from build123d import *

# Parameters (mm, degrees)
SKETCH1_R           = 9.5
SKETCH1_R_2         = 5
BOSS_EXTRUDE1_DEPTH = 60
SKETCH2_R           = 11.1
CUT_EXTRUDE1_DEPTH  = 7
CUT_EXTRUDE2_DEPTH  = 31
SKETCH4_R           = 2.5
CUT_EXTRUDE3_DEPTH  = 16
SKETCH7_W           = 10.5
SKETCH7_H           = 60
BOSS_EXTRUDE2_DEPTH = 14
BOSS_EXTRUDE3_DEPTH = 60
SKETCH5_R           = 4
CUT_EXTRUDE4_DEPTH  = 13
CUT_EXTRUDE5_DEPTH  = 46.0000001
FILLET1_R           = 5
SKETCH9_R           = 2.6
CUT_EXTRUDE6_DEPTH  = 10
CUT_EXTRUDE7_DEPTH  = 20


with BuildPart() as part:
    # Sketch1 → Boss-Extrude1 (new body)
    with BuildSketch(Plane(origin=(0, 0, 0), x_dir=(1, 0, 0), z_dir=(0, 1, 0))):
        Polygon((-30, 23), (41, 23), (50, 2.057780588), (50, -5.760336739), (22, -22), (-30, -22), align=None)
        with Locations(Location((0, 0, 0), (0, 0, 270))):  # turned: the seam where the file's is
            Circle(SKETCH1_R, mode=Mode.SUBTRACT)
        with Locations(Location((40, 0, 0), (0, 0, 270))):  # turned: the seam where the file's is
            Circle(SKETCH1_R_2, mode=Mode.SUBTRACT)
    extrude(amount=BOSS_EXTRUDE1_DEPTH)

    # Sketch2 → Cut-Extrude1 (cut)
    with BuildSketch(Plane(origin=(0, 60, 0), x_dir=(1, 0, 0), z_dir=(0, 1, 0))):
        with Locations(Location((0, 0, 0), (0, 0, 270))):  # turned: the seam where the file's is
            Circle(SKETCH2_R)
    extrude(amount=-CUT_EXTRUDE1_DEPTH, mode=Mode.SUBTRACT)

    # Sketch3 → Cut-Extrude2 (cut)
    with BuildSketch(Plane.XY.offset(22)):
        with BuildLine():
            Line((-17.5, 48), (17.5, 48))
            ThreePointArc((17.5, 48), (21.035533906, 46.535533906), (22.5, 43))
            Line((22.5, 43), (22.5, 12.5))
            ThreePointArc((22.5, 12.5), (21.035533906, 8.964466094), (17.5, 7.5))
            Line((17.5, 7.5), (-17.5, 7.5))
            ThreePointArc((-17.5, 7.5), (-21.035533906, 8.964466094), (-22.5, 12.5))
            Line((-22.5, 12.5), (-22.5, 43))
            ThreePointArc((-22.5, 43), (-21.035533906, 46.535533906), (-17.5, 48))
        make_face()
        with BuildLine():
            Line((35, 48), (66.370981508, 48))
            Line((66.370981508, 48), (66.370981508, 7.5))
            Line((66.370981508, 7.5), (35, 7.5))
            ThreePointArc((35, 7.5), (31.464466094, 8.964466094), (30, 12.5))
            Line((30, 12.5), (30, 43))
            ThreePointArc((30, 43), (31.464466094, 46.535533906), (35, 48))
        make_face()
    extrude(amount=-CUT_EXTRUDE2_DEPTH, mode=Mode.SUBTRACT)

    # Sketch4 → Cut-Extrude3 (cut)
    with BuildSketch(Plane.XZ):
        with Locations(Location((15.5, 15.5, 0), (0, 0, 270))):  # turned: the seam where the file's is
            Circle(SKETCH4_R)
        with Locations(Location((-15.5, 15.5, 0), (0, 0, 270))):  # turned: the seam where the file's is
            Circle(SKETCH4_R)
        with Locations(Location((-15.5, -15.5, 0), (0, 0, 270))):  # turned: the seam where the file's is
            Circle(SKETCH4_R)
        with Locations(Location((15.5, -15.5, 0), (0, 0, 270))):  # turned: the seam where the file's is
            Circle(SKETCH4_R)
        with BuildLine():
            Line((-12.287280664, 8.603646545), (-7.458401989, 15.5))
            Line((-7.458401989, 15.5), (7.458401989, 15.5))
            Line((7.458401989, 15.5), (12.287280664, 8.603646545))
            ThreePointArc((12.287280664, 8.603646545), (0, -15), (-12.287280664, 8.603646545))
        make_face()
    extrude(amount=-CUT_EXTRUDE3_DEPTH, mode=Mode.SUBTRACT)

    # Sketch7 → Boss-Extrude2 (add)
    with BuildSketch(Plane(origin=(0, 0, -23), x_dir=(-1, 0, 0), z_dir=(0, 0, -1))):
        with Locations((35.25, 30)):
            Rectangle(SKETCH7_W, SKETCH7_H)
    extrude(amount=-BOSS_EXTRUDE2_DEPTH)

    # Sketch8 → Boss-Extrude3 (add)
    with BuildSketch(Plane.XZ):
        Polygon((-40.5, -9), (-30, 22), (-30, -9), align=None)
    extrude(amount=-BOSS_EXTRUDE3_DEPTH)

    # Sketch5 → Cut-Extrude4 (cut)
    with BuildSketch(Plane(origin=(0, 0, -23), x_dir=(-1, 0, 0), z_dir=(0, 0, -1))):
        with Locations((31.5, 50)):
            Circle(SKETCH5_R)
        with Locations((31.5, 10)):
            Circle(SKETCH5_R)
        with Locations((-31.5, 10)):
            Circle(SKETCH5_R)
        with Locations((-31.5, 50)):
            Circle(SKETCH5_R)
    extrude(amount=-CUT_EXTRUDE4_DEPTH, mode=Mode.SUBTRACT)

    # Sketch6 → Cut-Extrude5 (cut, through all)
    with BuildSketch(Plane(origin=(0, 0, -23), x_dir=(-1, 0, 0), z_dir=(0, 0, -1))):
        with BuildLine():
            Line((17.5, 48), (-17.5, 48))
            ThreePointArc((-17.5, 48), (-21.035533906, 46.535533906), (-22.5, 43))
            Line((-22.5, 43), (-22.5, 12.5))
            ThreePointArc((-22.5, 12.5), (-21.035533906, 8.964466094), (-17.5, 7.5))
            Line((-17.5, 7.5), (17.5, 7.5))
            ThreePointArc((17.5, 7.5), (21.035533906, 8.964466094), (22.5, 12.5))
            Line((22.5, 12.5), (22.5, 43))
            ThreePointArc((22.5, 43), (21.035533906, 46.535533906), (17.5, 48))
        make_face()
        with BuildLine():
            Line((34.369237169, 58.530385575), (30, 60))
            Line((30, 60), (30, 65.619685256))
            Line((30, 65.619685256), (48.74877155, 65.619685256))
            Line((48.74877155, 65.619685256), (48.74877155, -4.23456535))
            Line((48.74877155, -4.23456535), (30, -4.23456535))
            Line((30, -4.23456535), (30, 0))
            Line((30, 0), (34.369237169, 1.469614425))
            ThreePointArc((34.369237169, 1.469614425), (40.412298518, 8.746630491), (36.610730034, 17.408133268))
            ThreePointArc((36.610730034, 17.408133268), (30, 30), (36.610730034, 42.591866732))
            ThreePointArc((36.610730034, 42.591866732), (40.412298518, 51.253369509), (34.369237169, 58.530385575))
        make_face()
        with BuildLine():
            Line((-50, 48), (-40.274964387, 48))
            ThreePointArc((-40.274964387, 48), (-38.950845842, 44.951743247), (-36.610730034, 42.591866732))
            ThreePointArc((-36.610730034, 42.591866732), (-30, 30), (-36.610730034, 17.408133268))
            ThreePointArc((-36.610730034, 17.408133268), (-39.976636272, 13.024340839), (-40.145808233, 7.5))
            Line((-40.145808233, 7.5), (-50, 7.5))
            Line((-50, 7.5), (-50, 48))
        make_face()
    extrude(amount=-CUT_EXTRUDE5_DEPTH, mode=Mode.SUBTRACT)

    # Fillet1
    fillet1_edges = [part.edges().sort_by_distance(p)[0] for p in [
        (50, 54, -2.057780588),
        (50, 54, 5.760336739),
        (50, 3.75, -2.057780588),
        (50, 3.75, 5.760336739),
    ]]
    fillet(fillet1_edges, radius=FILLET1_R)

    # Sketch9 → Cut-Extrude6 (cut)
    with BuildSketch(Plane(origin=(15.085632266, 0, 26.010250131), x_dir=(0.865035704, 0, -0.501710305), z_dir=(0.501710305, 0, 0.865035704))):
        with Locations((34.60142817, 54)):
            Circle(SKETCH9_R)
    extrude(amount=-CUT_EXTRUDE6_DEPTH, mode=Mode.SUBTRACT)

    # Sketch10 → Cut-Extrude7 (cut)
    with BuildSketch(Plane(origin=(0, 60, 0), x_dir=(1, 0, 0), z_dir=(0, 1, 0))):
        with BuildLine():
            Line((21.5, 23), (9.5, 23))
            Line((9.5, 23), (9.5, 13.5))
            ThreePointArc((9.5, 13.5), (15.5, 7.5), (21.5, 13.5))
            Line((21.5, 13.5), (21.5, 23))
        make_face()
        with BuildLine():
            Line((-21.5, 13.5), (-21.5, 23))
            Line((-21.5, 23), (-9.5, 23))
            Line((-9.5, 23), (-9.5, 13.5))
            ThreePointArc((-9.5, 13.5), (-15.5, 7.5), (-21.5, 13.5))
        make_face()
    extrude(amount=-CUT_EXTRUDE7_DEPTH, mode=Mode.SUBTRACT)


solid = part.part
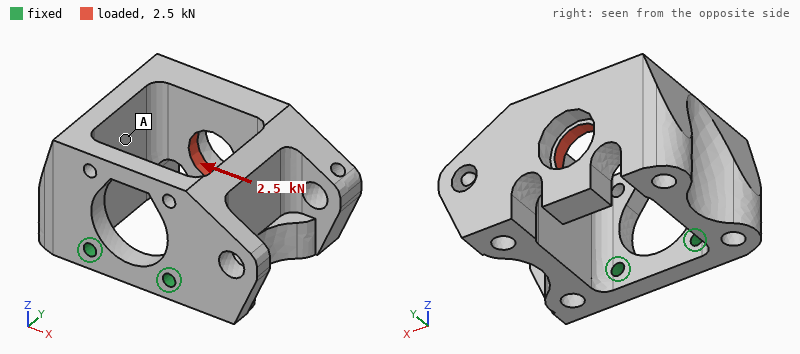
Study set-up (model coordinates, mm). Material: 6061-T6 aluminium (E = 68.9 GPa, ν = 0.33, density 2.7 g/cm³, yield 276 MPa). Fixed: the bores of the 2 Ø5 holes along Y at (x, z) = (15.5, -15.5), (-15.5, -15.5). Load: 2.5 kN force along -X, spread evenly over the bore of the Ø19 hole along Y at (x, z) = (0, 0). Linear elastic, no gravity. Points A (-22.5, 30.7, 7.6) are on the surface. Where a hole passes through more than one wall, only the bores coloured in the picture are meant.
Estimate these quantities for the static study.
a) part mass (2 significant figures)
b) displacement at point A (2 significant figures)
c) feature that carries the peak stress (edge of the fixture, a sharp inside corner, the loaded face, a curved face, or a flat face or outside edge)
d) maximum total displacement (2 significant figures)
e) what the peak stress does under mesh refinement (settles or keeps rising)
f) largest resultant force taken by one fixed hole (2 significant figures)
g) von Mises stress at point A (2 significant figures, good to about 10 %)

240 g
0.16 mm
edge of the fixture
0.31 mm
keeps rising
2.3 kN
22 MPa
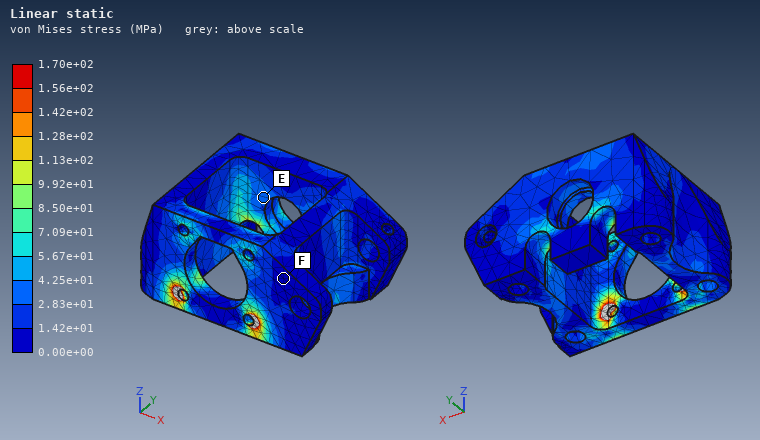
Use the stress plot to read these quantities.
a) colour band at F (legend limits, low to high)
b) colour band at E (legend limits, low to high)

0.00e+00 to 1.42e+01 MPa
2.83e+01 to 4.25e+01 MPa
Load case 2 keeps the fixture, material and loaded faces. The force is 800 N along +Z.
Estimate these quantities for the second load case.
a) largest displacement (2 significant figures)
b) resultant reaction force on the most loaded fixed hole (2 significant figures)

0.17 mm
410 N
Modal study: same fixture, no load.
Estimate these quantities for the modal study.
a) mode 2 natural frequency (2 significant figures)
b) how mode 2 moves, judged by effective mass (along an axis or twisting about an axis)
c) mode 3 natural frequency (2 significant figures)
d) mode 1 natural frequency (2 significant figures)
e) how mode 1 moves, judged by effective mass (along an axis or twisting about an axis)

1300 Hz
along X
2200 Hz
1000 Hz
along Z
